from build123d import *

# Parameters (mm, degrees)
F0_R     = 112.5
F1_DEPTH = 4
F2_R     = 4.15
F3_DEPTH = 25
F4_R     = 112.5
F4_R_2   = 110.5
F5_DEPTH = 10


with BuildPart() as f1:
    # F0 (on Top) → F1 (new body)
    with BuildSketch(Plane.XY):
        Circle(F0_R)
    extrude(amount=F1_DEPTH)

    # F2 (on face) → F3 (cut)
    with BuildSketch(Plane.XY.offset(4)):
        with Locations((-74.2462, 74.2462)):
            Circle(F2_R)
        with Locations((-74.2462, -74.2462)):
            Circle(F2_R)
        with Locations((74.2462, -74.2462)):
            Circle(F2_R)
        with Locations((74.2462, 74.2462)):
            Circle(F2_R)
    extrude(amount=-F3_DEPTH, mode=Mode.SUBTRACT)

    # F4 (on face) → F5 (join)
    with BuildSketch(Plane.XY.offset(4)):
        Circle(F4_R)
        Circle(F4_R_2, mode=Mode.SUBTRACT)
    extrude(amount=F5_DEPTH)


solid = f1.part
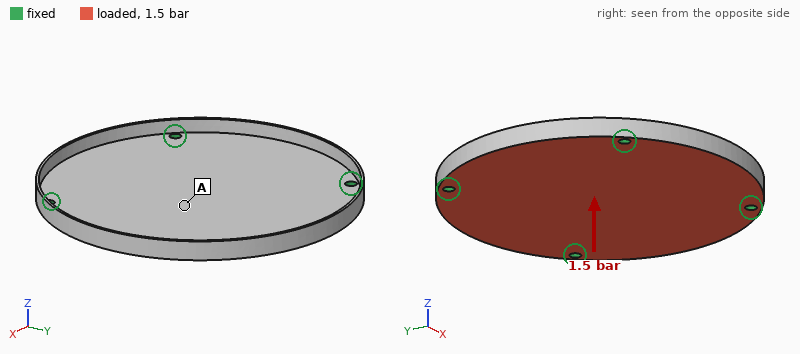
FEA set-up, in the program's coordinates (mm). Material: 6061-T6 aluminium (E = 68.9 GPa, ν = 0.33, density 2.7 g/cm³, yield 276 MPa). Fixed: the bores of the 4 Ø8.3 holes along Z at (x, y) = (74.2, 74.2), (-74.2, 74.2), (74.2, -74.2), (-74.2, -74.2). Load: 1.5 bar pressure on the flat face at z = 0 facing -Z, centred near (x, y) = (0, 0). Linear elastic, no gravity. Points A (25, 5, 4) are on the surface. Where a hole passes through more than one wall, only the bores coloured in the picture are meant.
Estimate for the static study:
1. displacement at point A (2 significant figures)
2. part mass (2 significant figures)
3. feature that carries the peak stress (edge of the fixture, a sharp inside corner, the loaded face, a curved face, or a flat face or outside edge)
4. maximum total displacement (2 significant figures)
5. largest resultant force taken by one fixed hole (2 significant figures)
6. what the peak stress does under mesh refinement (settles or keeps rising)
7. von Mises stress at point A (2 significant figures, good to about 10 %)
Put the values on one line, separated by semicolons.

1.0 mm; 460 g; edge of the fixture; 1.1 mm; 1.5 kN; keeps rising; 57 MPa
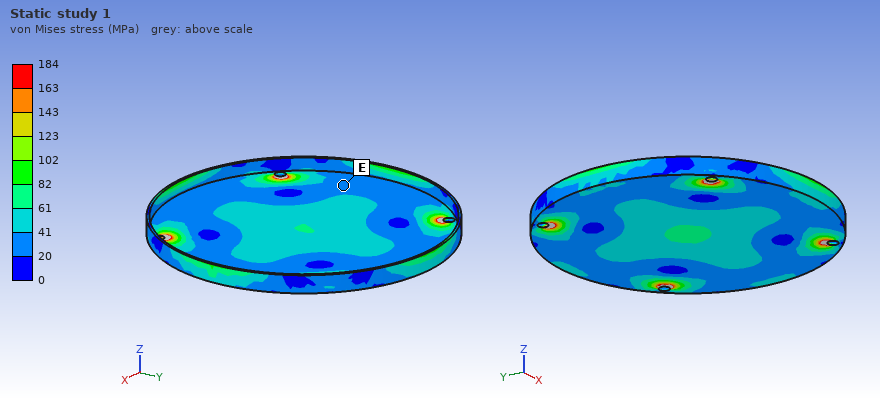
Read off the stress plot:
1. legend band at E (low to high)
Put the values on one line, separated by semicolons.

20 to 41 MPa
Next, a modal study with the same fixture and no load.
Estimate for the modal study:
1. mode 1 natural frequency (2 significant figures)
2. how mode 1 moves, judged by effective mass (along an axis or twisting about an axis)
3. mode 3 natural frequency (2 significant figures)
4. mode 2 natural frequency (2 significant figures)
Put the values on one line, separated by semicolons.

710 Hz; along Z; 1300 Hz; 1200 Hz
